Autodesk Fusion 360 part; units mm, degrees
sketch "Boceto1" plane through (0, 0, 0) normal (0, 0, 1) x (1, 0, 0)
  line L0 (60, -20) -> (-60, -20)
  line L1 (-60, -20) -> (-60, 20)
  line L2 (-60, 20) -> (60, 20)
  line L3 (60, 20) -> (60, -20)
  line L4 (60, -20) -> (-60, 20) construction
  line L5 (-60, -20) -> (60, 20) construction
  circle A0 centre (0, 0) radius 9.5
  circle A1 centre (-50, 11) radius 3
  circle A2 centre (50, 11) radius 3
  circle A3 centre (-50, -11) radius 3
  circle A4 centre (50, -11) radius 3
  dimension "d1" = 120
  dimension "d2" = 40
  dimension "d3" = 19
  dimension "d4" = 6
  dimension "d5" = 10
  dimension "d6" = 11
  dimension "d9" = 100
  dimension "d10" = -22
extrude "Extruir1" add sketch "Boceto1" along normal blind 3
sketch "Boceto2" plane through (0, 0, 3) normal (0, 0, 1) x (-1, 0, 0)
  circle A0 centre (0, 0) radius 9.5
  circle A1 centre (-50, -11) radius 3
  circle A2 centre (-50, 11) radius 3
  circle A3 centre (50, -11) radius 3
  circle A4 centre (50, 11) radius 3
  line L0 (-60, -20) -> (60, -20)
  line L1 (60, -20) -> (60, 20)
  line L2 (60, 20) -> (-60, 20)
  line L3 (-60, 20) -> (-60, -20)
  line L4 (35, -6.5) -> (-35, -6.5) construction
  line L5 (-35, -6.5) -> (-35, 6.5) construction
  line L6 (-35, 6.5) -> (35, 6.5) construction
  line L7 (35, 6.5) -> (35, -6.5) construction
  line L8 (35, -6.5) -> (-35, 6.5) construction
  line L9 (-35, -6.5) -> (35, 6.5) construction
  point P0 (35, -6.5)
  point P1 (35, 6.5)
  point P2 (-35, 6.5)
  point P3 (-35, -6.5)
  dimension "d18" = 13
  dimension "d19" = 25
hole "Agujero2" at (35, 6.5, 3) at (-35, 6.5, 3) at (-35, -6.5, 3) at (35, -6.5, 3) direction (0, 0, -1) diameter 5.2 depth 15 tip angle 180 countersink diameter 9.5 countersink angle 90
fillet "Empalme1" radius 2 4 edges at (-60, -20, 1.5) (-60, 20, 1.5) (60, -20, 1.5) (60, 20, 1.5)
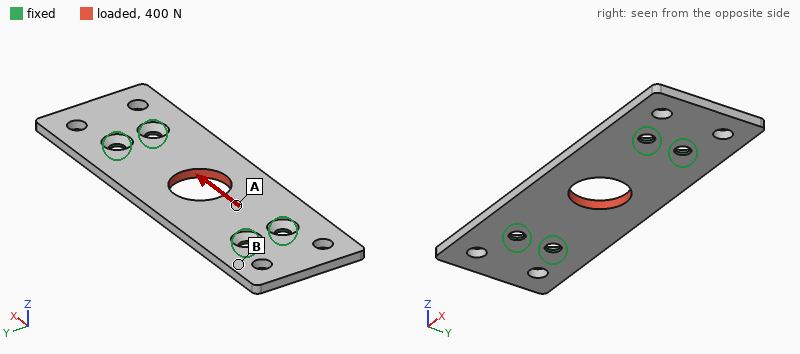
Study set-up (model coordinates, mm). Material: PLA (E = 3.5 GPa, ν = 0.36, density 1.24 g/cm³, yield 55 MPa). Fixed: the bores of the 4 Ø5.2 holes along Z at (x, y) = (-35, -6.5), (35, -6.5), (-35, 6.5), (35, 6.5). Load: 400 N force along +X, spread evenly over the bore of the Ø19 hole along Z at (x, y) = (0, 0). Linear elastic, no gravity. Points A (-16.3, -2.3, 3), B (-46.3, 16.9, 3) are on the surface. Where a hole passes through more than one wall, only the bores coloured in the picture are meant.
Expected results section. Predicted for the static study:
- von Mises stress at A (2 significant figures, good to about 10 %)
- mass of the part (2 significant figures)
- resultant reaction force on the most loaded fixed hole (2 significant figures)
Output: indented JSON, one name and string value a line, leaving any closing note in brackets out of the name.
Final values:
{
  "von Mises stress at A": "2.1 MPa",
  "mass of the part": "16 g",
  "resultant reaction force on the most loaded fixed hole": "100 N"
}
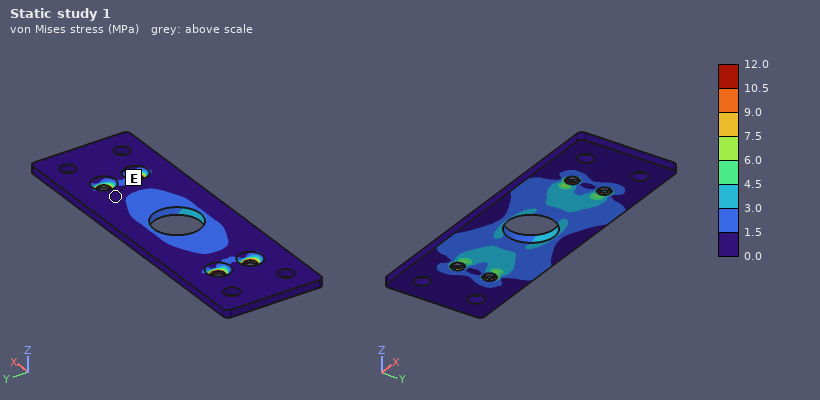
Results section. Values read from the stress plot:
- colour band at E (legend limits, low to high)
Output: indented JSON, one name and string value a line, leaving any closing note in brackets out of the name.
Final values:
{
  "colour band at E": "0.0 to 1.5 MPa"
}
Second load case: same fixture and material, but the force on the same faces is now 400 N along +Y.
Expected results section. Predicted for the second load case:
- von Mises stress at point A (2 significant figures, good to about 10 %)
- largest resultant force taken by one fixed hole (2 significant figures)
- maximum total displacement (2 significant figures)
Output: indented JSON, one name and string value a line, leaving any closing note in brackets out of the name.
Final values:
{
  "von Mises stress at point A": "4.4 MPa",
  "largest resultant force taken by one fixed hole": "140 N",
  "maximum total displacement": "84 µm"
}
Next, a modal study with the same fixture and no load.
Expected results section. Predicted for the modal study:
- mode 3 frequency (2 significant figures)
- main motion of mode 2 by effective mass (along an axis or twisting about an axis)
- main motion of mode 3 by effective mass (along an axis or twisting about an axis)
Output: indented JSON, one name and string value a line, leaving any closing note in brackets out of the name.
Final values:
{
  "mode 3 frequency": "1200 Hz",
  "main motion of mode 2 by effective mass": "twisting about Y",
  "main motion of mode 3 by effective mass": "along Z"
}
